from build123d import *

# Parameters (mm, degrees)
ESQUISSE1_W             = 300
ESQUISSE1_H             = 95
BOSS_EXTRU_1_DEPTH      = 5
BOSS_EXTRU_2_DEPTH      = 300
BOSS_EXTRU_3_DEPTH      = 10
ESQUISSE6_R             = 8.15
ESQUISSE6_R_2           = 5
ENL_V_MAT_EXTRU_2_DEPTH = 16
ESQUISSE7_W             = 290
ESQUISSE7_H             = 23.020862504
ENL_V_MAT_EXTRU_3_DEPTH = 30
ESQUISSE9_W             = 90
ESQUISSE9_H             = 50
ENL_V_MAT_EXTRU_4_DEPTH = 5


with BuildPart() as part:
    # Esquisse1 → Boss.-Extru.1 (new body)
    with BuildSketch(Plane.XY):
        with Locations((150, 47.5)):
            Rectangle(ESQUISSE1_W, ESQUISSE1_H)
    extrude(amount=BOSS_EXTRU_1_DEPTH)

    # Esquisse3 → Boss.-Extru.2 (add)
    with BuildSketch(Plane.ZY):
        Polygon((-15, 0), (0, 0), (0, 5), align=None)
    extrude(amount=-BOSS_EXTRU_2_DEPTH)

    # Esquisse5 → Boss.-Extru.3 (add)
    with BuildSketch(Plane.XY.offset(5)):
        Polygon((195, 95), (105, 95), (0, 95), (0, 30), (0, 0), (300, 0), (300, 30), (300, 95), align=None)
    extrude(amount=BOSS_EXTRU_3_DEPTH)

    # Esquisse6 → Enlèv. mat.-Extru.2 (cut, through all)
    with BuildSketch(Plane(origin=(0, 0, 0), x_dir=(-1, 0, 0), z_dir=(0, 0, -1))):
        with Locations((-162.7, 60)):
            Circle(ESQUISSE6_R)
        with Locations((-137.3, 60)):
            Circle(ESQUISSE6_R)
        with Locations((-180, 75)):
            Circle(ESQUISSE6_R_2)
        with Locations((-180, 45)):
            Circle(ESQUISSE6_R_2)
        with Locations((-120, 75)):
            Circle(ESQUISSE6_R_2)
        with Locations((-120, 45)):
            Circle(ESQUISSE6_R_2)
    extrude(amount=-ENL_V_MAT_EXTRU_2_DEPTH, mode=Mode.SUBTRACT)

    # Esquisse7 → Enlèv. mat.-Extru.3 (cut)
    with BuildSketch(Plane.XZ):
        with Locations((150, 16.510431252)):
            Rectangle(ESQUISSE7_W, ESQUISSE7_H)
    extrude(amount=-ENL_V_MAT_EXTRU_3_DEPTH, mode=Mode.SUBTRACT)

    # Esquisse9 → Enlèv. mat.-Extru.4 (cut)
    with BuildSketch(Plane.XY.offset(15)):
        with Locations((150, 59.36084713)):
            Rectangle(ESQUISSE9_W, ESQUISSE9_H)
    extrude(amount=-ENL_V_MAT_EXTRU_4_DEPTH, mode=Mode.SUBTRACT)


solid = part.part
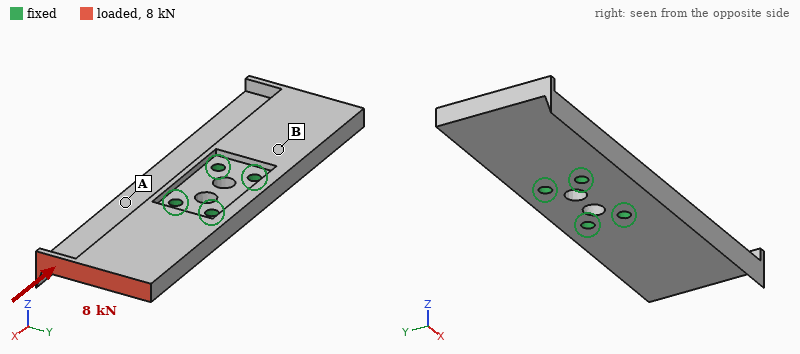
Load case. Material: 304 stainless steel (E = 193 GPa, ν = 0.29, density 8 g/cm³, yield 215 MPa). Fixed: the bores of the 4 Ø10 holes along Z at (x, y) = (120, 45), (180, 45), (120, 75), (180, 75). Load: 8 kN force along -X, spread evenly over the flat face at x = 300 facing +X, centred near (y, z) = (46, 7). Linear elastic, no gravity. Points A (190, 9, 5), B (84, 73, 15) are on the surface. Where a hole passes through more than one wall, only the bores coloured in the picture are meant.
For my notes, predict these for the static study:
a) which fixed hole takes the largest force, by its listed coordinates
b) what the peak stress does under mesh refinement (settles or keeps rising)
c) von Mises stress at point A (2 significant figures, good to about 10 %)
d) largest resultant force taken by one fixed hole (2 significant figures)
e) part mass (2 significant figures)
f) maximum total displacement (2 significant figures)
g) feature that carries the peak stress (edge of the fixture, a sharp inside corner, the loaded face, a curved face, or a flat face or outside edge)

(180, 45)
keeps rising
10 MPa
5.0 kN
2.6 kg
56 µm
edge of the fixture
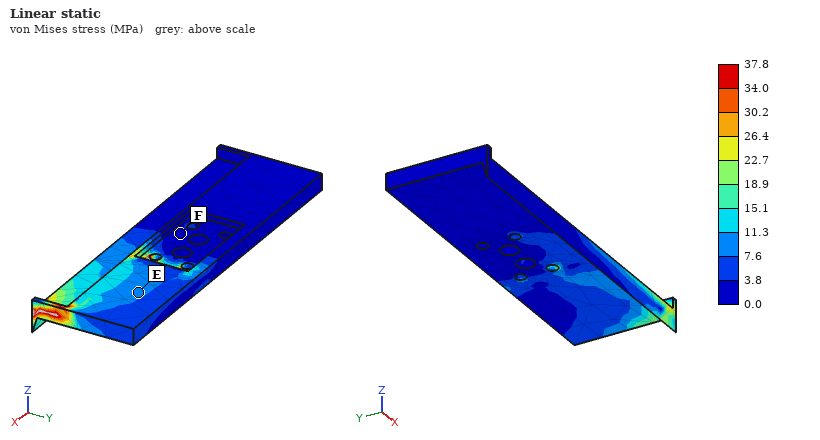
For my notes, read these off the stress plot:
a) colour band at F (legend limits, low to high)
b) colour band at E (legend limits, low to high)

0.0 to 3.8 MPa
7.6 to 11.3 MPa
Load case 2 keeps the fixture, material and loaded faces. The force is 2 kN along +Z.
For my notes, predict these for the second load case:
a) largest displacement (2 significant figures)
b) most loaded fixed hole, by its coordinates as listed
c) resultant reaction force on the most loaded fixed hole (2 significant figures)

0.45 mm
(180, 45)
3.5 kN
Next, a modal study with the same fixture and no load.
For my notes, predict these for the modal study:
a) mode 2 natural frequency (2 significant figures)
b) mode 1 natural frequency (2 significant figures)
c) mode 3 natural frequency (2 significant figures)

640 Hz
640 Hz
1800 Hz
